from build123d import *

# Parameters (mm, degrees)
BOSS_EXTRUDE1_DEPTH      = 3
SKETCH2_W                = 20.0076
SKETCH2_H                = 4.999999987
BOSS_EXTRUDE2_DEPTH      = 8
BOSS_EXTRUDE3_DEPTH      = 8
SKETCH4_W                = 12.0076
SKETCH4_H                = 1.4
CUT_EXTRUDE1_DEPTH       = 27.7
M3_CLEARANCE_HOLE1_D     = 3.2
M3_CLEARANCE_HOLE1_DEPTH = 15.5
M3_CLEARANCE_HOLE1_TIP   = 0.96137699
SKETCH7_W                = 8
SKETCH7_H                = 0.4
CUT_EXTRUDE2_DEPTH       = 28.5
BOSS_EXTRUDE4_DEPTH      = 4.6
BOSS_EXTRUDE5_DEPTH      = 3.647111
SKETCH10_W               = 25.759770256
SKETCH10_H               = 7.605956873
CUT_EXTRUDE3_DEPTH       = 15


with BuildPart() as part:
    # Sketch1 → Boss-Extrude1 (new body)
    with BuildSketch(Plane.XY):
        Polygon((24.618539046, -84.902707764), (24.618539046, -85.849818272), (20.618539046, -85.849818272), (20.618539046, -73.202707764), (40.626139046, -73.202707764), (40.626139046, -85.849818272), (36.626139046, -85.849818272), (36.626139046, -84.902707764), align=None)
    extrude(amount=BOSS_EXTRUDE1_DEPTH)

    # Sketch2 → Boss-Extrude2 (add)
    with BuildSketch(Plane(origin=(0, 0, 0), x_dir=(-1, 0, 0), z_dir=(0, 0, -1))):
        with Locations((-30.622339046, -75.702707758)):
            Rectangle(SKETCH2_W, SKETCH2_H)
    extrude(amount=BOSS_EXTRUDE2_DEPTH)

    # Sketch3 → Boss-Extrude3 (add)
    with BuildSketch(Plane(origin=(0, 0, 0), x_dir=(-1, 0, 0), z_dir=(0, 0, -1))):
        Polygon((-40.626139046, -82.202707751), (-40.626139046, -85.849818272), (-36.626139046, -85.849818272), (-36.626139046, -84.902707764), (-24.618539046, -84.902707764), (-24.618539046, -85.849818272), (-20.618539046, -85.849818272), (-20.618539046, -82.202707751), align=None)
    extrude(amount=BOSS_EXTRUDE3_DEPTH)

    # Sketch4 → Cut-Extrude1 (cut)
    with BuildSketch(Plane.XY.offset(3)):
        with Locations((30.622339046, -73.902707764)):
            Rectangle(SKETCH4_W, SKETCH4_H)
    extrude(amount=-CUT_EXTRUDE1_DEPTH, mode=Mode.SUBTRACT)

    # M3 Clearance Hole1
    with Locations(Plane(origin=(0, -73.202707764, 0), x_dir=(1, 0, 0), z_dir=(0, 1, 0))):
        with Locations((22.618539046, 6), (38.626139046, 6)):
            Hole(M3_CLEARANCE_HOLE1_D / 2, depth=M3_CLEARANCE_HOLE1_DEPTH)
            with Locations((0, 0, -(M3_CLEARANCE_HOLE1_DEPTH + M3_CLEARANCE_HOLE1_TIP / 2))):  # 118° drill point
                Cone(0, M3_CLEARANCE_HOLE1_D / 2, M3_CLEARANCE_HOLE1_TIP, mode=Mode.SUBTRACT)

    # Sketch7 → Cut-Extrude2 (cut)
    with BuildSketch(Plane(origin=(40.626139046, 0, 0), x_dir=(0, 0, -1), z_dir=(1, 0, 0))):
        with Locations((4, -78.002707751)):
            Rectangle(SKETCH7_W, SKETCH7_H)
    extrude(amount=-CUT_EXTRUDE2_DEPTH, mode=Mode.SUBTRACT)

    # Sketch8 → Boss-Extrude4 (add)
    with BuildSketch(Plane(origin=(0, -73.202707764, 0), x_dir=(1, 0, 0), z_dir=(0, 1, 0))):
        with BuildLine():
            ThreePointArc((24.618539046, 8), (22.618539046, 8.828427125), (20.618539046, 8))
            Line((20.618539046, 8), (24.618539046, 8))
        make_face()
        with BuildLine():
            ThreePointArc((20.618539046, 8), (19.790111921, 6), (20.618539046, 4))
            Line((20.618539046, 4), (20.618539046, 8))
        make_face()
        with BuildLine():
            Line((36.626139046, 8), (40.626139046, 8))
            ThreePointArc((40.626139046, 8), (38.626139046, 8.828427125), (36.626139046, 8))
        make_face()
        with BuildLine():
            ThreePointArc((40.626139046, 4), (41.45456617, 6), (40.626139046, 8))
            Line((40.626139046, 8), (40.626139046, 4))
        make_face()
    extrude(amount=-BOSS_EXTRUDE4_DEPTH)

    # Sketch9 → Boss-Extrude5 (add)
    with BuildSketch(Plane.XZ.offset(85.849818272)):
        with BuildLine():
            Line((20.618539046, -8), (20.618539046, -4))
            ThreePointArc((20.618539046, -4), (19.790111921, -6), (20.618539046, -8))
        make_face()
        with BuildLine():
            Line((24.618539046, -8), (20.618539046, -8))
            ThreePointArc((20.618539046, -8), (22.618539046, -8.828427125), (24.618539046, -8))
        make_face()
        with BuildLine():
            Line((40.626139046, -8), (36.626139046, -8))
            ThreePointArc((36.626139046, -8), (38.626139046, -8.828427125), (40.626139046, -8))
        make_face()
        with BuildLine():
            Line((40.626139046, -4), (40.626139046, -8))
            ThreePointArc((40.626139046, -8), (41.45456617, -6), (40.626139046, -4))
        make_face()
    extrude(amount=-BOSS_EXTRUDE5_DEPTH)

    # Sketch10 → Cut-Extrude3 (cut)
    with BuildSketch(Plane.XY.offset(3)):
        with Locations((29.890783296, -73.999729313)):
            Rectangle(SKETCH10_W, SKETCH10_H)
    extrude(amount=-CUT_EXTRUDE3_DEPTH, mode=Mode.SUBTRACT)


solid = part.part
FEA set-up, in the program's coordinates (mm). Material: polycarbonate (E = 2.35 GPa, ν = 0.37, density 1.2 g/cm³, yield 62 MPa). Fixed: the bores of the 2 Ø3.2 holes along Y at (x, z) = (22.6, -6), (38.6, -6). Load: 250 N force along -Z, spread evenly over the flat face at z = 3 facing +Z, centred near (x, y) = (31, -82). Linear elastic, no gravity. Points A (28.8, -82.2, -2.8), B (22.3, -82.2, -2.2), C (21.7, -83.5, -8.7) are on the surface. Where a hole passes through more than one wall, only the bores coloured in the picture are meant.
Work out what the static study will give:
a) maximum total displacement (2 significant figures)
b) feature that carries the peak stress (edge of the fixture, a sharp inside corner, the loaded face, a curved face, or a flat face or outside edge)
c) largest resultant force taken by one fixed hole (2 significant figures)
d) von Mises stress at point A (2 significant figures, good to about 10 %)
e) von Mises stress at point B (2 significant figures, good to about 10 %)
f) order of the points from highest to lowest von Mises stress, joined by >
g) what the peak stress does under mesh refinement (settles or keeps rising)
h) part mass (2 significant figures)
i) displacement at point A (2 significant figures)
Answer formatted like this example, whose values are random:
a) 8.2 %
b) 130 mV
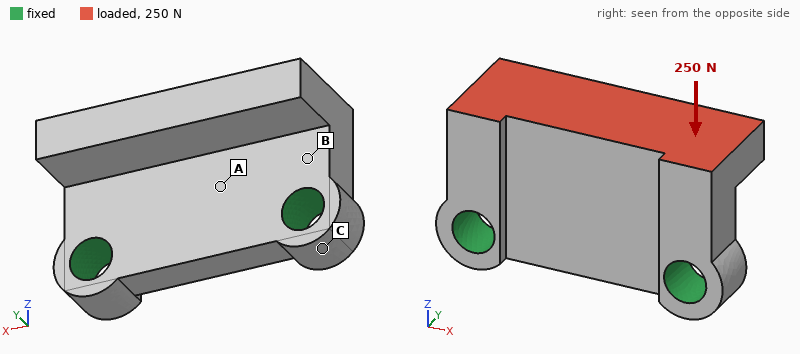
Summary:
a) 0.28 mm
b) edge of the fixture
c) 130 N
d) 12 MPa
e) 25 MPa
f) B > A > C
g) keeps rising
h) 1.1 g
i) 0.048 mm
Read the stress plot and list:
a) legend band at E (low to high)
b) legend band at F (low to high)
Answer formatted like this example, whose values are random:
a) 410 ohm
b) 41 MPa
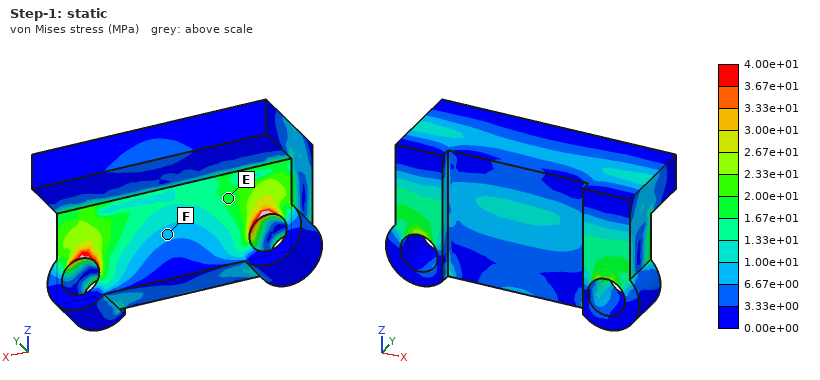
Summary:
a) 1.67e+01 to 2.00e+01 MPa
b) 6.67e+00 to 1.00e+01 MPa
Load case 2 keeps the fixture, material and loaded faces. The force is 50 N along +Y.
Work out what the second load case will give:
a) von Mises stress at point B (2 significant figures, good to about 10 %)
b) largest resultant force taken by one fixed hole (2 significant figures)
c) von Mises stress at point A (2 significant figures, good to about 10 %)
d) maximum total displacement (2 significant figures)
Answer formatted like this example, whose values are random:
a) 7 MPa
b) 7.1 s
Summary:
a) 9.8 MPa
b) 25 N
c) 3.9 MPa
d) 0.13 mm
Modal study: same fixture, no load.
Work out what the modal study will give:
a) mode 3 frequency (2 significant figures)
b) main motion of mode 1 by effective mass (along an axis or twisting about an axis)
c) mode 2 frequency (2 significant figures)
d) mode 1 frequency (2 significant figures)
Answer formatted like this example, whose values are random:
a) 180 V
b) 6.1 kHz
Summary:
a) 14 kHz
b) along Y
c) 8800 Hz
d) 5400 Hz
